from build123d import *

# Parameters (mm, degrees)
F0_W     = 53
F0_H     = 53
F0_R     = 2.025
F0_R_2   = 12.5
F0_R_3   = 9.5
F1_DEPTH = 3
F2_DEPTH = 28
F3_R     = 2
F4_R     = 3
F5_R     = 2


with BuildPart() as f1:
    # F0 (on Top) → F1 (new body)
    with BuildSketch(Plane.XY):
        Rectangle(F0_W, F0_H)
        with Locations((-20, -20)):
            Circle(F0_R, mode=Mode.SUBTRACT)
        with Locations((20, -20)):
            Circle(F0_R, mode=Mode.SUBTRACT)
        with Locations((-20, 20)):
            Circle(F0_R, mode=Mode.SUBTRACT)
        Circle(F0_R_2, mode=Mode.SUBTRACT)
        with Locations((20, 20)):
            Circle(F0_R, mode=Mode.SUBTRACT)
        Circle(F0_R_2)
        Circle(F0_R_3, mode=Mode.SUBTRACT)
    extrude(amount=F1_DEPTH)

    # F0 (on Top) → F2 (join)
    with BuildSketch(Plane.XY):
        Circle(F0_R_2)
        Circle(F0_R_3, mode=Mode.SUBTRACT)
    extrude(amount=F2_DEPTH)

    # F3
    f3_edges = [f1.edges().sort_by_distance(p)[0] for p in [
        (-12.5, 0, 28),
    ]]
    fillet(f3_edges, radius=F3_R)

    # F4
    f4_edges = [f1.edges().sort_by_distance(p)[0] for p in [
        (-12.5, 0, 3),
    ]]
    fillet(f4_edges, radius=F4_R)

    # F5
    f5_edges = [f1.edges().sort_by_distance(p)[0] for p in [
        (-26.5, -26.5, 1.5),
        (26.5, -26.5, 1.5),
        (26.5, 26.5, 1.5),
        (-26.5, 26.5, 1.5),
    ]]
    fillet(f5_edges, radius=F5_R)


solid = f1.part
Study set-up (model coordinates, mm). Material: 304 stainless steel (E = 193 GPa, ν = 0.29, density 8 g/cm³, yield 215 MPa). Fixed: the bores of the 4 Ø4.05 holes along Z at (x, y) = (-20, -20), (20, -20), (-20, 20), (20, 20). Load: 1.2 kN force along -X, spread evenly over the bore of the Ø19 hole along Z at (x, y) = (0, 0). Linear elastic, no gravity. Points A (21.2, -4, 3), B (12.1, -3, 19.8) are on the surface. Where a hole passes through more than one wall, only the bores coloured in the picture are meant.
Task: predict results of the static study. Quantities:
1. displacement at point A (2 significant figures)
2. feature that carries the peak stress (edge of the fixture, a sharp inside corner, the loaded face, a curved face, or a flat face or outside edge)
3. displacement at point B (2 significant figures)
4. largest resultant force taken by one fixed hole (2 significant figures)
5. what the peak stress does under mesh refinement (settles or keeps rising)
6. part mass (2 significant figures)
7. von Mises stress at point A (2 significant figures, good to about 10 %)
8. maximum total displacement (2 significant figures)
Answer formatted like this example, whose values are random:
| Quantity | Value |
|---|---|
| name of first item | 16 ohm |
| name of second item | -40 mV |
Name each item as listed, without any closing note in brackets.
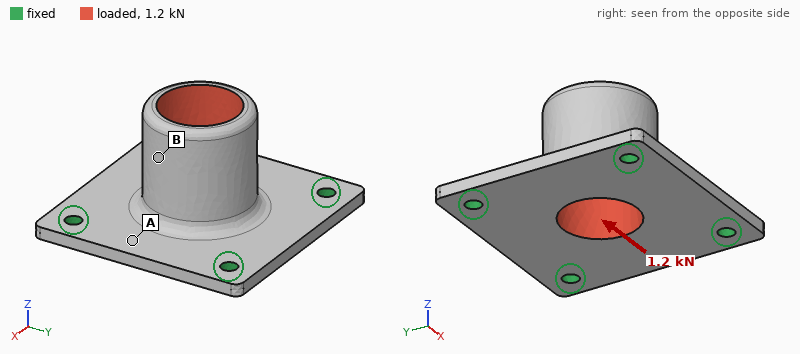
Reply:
| Quantity | Value |
|---|---|
| displacement at point A | 8.0 µm |
| feature that carries the peak stress | edge of the fixture |
| displacement at point B | 17 µm |
| largest resultant force taken by one fixed hole | 400 N |
| what the peak stress does under mesh refinement | keeps rising |
| part mass | 100 g |
| von Mises stress at point A | 19 MPa |
| maximum total displacement | 22 µm |
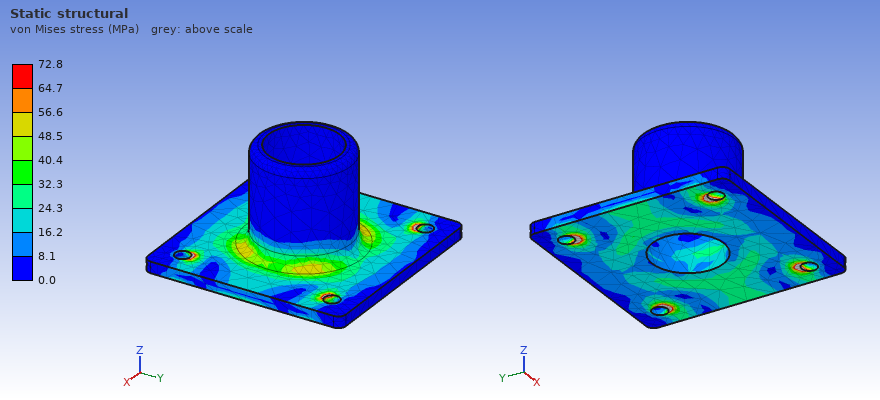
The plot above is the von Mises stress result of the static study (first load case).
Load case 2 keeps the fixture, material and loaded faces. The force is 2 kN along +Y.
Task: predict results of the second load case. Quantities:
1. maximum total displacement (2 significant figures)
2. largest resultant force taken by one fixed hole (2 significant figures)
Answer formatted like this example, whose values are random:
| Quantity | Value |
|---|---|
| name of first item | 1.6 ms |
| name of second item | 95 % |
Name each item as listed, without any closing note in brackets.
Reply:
| Quantity | Value |
|---|---|
| maximum total displacement | 37 µm |
| largest resultant force taken by one fixed hole | 670 N |
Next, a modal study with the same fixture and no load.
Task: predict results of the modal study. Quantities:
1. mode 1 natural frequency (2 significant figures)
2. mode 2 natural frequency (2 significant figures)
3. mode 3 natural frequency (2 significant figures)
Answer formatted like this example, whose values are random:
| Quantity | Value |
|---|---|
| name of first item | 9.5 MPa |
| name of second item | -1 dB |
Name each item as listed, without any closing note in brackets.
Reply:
| Quantity | Value |
|---|---|
| mode 1 natural frequency | 5800 Hz |
| mode 2 natural frequency | 5800 Hz |
| mode 3 natural frequency | 5800 Hz |
